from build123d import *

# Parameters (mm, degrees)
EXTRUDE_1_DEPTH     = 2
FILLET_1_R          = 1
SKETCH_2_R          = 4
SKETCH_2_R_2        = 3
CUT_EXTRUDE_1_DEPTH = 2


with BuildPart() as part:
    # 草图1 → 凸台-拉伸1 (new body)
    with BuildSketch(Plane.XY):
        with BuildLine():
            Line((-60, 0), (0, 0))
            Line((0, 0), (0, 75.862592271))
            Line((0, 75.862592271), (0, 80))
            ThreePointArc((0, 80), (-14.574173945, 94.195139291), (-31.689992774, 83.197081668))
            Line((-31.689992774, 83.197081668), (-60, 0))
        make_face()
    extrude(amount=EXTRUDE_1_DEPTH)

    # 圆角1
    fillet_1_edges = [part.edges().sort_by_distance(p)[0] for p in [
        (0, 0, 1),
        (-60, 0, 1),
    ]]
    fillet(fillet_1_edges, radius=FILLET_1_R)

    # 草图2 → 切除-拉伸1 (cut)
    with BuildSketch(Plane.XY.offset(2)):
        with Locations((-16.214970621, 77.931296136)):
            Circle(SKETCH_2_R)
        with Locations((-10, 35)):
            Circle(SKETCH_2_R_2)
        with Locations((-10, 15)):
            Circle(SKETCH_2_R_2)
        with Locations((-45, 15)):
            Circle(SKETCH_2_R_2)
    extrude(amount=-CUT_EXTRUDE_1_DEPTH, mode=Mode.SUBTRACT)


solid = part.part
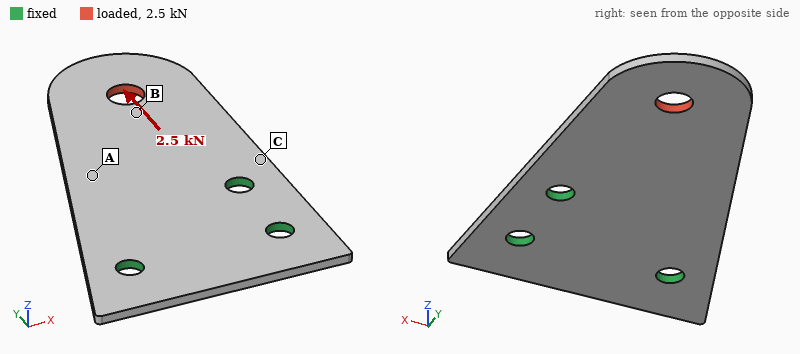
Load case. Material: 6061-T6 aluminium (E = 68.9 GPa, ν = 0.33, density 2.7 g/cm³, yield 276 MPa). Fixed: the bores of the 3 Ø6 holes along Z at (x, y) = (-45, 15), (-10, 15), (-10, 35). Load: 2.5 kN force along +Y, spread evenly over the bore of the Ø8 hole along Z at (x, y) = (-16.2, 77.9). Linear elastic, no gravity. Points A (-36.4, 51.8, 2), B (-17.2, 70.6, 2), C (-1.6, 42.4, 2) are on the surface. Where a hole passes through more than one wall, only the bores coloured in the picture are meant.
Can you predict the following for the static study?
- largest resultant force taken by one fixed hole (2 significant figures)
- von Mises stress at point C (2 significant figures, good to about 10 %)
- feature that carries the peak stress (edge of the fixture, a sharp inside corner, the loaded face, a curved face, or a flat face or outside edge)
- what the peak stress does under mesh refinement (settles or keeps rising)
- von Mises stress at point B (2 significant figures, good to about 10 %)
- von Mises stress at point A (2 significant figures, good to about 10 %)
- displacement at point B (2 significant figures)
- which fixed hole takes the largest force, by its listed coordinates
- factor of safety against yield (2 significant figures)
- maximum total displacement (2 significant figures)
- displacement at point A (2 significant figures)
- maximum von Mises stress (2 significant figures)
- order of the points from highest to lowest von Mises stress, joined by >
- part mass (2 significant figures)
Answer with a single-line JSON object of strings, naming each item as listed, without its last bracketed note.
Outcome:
{"largest resultant force taken by one fixed hole": "1.6 kN", "von Mises stress at point C": "36 MPa", "feature that carries the peak stress": "the loaded face", "what the peak stress does under mesh refinement": "settles", "von Mises stress at point B": "53 MPa", "von Mises stress at point A": "14 MPa", "displacement at point B": "23 µm", "which fixed hole takes the largest force, by its listed coordinates": "(-10, 35)", "factor of safety against yield": "2.4", "maximum total displacement": "35 µm", "displacement at point A": "7.3 µm", "maximum von Mises stress": "110 MPa", "order of the points from highest to lowest von Mises stress, joined by >": "B > C > A", "part mass": "21 g"}
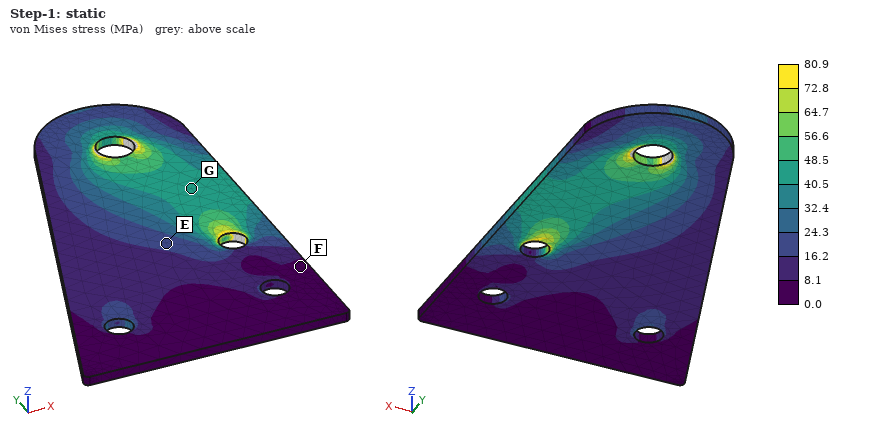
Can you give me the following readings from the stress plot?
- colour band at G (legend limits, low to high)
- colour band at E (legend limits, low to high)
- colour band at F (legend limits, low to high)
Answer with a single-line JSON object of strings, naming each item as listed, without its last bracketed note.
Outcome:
{"colour band at G": "40.5 to 48.5 MPa", "colour band at E": "16.2 to 24.3 MPa", "colour band at F": "0.0 to 8.1 MPa"}
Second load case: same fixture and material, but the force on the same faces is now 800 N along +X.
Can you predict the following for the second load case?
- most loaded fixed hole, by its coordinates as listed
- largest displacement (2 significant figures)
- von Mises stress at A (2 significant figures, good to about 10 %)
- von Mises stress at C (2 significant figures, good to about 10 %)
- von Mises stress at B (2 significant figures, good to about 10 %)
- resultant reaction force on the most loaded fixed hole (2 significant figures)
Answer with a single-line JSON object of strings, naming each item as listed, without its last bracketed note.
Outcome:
{"most loaded fixed hole, by its coordinates as listed": "(-10, 35)", "largest displacement": "72 µm", "von Mises stress at A": "31 MPa", "von Mises stress at C": "37 MPa", "von Mises stress at B": "35 MPa", "resultant reaction force on the most loaded fixed hole": "1.1 kN"}
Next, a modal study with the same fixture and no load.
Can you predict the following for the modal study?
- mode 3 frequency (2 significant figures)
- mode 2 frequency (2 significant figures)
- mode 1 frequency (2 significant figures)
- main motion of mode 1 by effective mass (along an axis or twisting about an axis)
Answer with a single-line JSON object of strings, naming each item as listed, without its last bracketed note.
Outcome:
{"mode 3 frequency": "3000 Hz", "mode 2 frequency": "1700 Hz", "mode 1 frequency": "580 Hz", "main motion of mode 1 by effective mass": "along Z"}
